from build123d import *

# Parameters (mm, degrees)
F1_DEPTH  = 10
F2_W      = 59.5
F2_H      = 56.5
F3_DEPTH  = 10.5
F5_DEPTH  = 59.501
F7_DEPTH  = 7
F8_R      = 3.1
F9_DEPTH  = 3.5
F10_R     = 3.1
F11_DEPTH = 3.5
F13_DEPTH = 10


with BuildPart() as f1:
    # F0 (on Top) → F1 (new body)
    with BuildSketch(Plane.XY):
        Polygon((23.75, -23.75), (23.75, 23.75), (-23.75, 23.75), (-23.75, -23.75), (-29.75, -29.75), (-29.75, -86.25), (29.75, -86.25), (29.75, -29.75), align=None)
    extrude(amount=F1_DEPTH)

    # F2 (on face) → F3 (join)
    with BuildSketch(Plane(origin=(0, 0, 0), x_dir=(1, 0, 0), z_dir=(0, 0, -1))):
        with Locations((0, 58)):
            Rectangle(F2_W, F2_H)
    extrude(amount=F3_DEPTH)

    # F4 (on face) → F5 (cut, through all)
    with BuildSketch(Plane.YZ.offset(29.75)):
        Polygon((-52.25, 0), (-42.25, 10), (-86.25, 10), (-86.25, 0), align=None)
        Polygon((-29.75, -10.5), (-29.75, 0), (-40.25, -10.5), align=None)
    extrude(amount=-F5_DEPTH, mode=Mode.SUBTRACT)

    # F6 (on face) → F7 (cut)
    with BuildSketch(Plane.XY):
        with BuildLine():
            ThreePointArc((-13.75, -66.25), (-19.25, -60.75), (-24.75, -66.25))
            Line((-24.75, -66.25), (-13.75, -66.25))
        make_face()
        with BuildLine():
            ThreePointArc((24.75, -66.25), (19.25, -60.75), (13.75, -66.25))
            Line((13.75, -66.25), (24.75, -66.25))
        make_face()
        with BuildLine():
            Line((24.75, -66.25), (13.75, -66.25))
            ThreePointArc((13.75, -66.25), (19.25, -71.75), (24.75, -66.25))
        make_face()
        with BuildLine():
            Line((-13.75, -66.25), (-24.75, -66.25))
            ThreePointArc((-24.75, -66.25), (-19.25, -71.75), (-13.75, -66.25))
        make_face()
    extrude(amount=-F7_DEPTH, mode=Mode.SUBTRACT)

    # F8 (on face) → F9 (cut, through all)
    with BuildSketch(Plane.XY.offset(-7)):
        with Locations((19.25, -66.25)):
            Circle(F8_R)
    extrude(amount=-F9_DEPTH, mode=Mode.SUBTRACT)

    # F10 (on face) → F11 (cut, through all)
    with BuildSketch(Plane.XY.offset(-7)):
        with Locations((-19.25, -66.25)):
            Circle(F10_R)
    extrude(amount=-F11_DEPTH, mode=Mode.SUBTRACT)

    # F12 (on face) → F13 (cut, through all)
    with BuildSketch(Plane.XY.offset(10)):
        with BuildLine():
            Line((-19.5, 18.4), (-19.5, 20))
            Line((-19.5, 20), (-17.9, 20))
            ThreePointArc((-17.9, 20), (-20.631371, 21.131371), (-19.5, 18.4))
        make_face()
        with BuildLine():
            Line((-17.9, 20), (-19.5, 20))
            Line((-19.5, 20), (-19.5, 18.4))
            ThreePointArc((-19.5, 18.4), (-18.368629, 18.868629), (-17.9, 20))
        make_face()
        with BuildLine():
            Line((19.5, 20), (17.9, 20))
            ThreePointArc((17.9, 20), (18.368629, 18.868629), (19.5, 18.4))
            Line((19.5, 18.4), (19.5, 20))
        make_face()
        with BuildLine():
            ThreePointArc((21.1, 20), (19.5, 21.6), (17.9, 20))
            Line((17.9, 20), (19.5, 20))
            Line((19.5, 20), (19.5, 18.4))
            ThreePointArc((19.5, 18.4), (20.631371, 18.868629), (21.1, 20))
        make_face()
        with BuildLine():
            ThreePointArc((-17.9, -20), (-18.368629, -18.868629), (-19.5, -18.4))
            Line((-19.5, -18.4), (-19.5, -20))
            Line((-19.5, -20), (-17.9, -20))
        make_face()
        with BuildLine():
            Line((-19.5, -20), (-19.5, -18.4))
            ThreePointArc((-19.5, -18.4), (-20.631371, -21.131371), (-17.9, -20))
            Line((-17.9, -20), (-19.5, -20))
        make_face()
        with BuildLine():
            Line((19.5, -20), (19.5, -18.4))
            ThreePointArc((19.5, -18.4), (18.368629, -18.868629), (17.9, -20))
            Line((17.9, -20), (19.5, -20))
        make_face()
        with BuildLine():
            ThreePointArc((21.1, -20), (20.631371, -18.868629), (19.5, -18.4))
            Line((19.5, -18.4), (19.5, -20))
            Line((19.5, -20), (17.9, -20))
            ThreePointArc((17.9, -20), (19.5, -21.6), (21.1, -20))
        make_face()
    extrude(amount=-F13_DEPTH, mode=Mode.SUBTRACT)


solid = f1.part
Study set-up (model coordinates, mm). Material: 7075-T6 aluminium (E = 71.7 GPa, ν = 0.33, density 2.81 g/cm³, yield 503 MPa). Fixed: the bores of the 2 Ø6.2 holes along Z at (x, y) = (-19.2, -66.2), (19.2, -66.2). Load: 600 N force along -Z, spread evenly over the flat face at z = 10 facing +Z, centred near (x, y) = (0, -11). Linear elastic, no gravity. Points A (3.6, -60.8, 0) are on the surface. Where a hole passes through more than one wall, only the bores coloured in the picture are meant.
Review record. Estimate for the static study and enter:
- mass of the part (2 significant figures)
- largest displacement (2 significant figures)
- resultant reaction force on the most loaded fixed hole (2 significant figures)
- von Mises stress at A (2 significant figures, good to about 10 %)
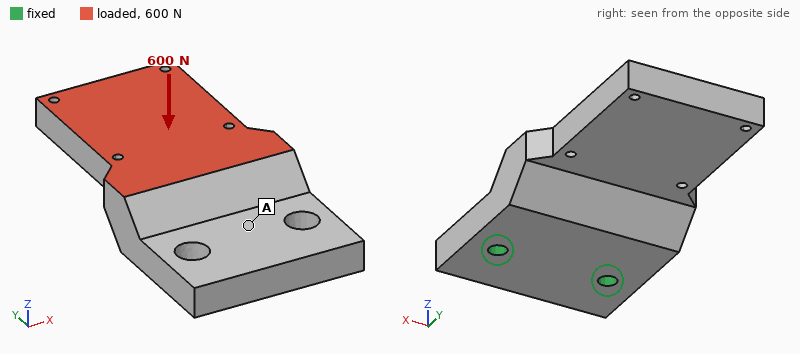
190 g
0.42 mm
350 N
24 MPa
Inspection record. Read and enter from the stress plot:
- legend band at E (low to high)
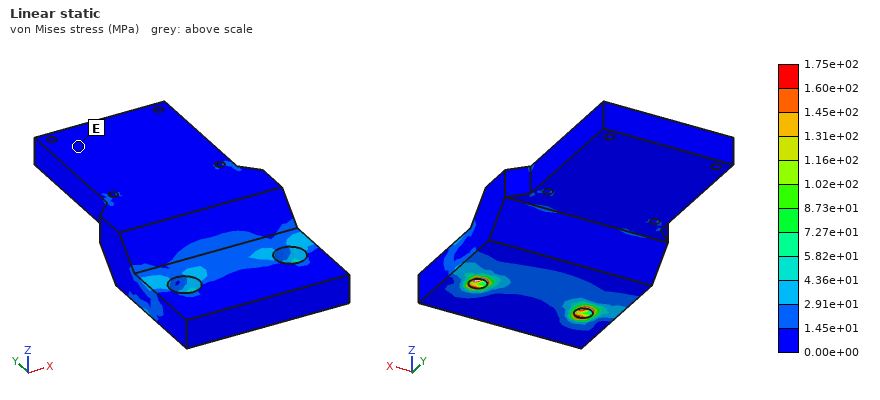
0.00e+00 to 1.45e+01 MPa
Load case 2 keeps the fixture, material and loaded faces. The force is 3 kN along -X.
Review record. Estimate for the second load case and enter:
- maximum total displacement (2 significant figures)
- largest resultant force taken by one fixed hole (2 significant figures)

74 µm
4.6 kN
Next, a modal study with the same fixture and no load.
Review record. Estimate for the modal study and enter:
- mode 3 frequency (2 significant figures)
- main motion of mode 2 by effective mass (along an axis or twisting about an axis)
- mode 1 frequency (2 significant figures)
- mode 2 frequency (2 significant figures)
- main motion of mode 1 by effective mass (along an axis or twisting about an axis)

4400 Hz
along X
740 Hz
3600 Hz
along Z
